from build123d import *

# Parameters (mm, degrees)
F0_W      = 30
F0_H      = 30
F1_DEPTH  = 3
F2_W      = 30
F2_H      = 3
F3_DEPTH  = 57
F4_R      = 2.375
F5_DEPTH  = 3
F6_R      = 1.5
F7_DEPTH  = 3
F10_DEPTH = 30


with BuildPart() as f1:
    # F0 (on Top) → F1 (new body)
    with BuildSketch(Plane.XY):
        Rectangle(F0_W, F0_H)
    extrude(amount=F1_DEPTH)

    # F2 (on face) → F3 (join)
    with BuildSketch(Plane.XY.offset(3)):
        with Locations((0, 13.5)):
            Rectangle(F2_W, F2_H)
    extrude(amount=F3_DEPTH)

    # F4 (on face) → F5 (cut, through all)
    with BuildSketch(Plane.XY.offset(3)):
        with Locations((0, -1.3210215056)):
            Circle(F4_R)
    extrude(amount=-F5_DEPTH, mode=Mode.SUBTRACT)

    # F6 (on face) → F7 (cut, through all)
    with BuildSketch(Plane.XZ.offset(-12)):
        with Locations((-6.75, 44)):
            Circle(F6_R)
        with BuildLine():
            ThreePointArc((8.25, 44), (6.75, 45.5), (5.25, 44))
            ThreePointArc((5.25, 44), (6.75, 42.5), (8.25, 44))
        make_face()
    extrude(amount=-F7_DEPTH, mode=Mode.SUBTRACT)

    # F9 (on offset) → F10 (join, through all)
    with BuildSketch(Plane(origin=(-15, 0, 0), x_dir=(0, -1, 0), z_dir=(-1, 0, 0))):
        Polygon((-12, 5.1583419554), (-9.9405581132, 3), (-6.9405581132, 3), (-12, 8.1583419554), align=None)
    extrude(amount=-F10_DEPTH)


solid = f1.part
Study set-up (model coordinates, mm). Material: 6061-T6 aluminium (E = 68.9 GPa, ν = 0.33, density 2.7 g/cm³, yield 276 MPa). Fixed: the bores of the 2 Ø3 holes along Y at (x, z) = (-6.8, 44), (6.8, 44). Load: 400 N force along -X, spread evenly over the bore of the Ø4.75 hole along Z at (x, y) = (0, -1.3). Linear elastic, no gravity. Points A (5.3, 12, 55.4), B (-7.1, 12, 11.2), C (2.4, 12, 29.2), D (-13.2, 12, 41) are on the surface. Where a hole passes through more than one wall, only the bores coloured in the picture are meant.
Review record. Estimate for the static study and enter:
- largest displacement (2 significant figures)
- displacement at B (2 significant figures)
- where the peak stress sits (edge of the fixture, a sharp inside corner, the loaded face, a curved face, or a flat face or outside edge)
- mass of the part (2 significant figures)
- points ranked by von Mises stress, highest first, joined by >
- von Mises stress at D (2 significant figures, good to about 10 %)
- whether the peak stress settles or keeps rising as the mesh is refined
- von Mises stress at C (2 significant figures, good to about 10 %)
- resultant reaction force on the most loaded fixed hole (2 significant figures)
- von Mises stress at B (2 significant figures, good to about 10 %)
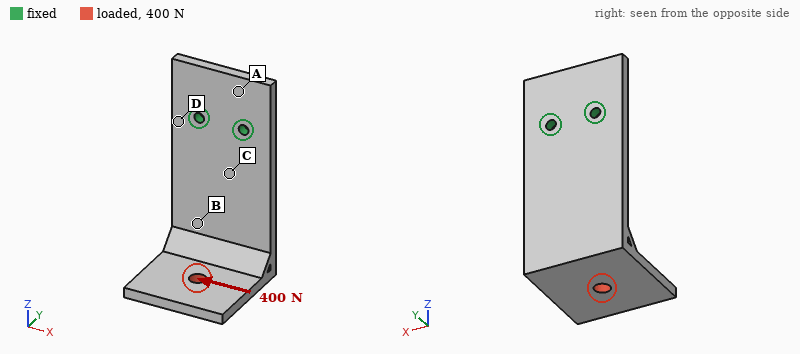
0.82 mm
0.17 mm
edge of the fixture
22 g
C > B > D > A
65 MPa
keeps rising
120 MPa
1.2 kN
89 MPa
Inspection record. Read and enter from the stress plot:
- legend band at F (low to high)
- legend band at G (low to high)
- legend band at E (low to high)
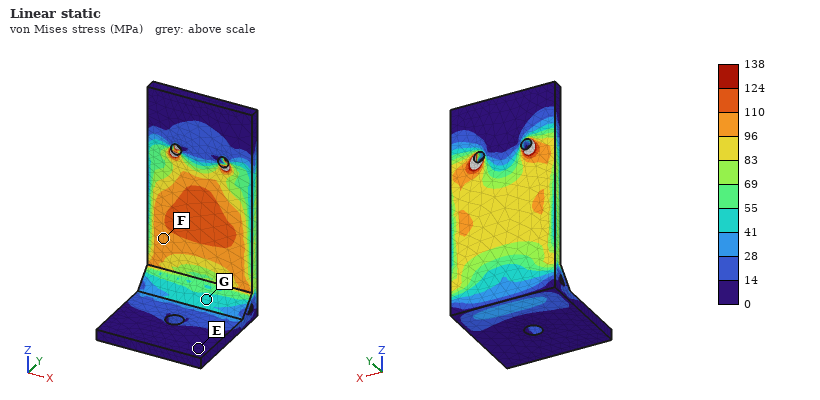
96 to 110 MPa
41 to 55 MPa
0 to 14 MPa
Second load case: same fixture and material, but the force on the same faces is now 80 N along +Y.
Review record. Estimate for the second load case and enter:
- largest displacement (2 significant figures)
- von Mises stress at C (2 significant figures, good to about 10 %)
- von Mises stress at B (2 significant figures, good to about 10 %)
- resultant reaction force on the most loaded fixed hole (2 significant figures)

0.61 mm
45 MPa
17 MPa
40 N
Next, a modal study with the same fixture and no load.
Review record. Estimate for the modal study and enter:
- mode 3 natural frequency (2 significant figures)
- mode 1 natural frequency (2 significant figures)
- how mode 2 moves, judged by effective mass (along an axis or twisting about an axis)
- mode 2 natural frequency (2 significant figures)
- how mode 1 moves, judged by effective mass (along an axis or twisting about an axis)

2600 Hz
620 Hz
along X
1500 Hz
along Y
